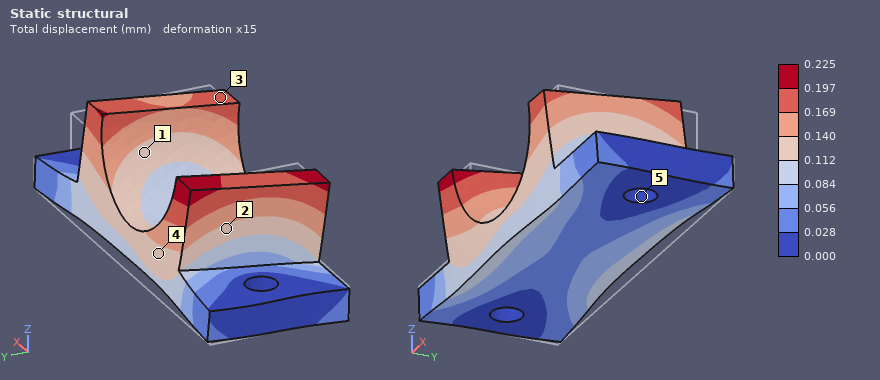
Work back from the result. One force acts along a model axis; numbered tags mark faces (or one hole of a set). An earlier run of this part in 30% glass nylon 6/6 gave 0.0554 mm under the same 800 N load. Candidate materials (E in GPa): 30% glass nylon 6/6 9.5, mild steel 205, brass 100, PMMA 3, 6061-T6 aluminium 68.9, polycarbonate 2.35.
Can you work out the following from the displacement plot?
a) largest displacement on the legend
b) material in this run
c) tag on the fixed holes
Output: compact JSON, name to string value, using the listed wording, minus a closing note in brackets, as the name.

{"largest displacement on the legend": "0.225 mm", "material in this run": "polycarbonate", "tag on the fixed holes": "5"}
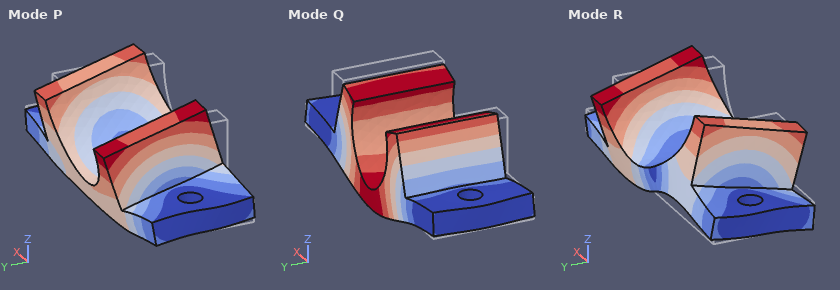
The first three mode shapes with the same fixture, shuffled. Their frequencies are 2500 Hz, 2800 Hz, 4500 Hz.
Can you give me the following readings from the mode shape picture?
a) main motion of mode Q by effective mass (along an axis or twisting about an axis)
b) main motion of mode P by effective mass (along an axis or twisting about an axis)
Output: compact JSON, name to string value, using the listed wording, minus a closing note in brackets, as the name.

{"main motion of mode Q by effective mass": "along Z", "main motion of mode P by effective mass": "along Y"}
